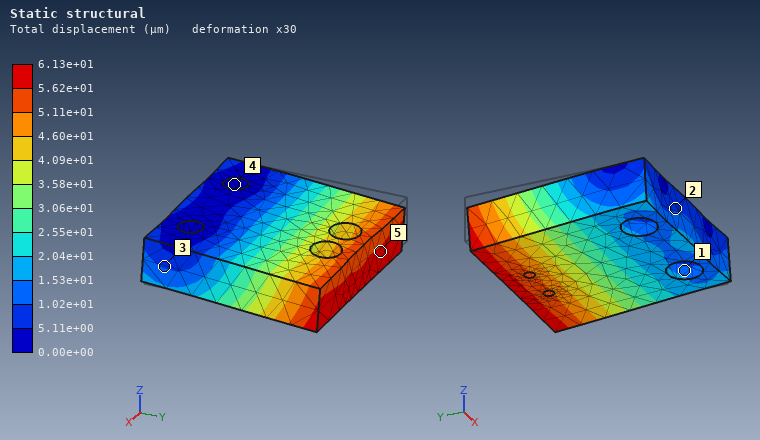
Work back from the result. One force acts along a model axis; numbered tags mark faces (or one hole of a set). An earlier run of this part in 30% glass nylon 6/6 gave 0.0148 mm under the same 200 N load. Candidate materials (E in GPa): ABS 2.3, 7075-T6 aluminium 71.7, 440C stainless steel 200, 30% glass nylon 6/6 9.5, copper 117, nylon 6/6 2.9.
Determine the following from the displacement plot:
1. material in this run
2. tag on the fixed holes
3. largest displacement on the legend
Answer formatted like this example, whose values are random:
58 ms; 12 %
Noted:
ABS; 4; 6.13e+01 µm
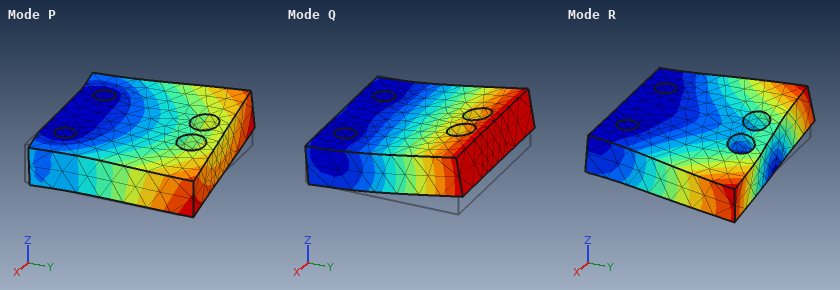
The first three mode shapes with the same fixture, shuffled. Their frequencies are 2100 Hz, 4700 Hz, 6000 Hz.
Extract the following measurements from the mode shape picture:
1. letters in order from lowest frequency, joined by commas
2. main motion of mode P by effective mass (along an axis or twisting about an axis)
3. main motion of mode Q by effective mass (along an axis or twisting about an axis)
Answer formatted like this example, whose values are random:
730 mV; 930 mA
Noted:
Q, R, P; along X; along Z
